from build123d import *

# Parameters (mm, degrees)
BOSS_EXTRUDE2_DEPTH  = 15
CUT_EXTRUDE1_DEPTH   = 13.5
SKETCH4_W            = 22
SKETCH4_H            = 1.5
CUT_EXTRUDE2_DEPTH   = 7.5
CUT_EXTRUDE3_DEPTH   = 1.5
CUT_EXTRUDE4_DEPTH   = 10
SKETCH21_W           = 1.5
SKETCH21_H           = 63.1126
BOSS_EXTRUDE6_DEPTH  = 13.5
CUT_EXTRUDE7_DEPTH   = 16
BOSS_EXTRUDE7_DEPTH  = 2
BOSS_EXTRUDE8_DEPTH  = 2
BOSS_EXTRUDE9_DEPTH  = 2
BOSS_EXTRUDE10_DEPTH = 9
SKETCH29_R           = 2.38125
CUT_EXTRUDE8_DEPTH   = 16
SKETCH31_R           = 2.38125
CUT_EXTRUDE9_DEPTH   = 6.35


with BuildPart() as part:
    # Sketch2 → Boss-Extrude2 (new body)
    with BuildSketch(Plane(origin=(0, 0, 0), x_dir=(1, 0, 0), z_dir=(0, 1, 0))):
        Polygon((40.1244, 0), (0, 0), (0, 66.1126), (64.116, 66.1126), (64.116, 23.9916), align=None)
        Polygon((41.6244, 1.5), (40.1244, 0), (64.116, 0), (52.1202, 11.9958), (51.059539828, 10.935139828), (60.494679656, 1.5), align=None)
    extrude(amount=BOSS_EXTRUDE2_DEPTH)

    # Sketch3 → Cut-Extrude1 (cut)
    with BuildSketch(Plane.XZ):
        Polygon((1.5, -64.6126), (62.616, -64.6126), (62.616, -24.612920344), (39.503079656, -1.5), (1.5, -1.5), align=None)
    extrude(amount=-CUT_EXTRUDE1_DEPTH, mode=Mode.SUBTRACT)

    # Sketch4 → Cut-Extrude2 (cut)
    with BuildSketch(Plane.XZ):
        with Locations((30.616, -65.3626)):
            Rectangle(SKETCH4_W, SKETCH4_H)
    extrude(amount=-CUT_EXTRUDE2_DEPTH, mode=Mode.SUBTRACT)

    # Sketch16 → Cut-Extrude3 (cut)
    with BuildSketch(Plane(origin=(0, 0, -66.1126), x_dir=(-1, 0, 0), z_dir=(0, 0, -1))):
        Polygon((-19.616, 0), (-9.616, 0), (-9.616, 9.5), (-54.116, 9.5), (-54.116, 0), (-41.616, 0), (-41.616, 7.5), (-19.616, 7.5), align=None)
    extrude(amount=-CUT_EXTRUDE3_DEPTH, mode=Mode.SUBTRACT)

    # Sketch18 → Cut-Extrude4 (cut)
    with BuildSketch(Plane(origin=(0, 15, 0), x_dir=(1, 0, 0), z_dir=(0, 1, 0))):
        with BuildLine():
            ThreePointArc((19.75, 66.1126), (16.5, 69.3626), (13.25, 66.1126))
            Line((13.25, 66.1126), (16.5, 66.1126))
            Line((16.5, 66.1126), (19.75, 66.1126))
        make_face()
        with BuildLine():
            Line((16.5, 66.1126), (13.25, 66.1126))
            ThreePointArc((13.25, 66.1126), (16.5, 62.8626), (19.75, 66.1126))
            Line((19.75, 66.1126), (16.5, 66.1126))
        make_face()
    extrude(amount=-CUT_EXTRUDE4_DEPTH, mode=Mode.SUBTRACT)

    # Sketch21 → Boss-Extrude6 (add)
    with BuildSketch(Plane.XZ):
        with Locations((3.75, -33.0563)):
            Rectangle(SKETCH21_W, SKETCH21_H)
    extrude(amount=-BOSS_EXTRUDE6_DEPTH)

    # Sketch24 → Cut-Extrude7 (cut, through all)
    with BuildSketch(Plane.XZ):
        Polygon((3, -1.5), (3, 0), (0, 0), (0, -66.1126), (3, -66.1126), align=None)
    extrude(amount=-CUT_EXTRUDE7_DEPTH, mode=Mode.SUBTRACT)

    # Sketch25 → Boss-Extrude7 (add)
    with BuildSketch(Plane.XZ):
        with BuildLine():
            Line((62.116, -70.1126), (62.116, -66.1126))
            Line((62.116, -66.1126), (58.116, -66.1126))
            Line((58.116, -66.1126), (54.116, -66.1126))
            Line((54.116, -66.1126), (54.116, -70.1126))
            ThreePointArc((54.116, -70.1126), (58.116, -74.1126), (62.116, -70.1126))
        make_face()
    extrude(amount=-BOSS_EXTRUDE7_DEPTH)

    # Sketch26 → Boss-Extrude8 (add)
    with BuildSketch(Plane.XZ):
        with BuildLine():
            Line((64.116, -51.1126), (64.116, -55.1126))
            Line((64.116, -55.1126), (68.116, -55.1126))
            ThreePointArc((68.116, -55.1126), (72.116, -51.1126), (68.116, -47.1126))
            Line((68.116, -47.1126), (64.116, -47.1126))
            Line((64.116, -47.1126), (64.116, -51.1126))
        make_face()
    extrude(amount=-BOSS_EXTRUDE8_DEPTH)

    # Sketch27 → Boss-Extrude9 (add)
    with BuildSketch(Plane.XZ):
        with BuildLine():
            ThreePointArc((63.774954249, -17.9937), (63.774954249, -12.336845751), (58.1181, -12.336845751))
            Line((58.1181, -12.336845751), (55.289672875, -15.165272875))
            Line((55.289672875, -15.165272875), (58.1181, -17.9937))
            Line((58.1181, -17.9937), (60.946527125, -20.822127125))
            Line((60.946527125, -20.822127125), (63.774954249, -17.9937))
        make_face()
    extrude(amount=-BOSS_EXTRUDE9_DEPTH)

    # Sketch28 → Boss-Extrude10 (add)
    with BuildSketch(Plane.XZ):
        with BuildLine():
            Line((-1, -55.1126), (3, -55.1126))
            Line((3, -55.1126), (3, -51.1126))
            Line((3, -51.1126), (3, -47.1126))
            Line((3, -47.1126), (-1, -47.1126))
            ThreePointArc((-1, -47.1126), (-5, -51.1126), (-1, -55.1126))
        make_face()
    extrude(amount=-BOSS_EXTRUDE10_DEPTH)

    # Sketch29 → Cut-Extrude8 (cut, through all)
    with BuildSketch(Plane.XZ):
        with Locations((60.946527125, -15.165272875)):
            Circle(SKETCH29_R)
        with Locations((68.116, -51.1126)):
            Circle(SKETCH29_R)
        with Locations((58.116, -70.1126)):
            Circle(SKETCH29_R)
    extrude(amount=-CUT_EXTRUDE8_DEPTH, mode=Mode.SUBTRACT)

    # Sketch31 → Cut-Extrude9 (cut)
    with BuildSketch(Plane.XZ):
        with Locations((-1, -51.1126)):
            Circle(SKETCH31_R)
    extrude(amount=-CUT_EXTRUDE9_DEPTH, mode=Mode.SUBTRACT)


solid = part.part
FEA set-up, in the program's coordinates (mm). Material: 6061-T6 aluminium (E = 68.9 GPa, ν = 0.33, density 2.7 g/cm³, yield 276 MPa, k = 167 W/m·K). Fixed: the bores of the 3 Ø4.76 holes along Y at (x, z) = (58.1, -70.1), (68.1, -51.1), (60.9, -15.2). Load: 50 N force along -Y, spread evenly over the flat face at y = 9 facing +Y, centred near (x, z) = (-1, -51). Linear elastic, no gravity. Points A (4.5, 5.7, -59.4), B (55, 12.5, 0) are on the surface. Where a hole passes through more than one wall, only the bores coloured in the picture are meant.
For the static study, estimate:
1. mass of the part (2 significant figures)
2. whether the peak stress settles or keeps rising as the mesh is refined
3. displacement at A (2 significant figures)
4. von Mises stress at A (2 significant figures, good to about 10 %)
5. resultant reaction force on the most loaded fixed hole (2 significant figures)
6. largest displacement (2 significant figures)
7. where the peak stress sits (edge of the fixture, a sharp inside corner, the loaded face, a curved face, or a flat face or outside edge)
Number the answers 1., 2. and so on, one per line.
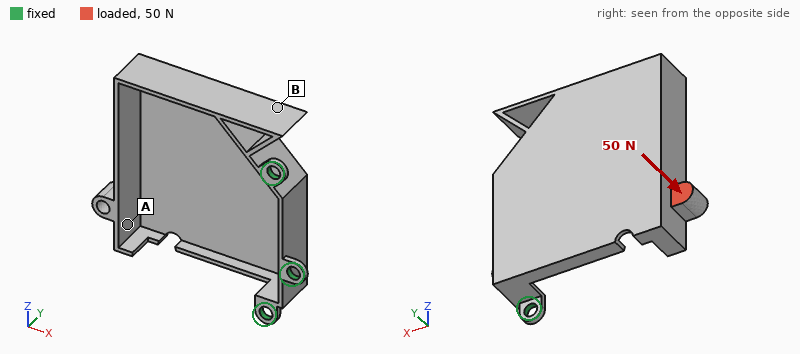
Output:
1. 30 g
2. keeps rising
3. 0.89 mm
4. 23 MPa
5. 230 N
6. 1.1 mm
7. a sharp inside corner
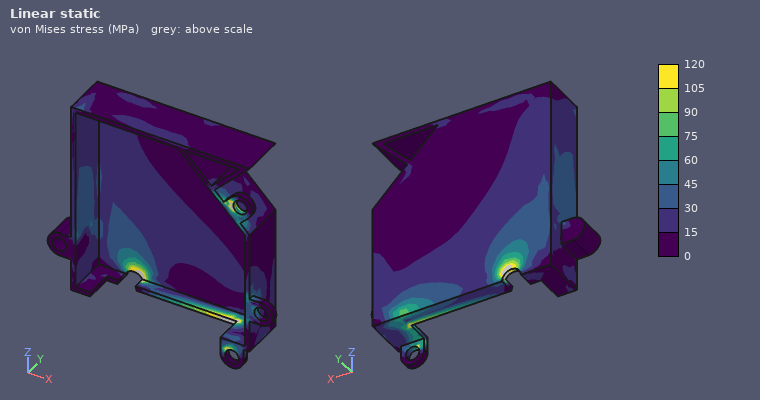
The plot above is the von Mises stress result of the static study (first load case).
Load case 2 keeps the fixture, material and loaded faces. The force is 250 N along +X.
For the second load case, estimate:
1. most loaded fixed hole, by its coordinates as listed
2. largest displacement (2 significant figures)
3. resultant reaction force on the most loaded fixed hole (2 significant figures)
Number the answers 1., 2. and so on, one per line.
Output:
1. (58.1, -70.1)
2. 0.69 mm
3. 200 N
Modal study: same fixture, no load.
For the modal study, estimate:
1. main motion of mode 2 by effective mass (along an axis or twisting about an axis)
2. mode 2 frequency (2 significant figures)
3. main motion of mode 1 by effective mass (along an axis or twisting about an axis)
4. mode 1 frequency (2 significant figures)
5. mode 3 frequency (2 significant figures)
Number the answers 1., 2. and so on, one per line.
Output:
1. along Z
2. 680 Hz
3. along Y
4. 460 Hz
5. 1600 Hz
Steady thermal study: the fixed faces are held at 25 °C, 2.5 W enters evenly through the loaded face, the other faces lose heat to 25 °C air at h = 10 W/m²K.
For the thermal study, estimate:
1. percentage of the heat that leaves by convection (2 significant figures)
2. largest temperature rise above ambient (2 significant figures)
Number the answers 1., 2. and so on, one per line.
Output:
1. 29 %
2. 14 K
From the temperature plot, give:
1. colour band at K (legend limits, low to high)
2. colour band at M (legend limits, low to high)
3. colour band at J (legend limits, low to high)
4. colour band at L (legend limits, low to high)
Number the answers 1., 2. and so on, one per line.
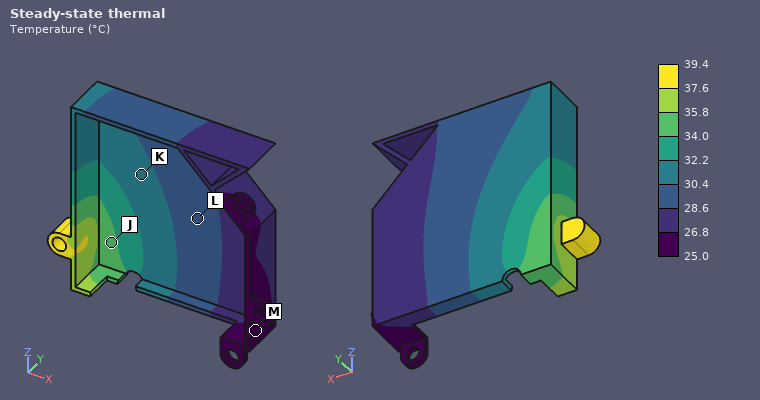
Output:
1. 30.4 to 32.2 °C
2. 25.0 to 26.8 °C
3. 34.0 to 35.8 °C
4. 28.6 to 30.4 °C
